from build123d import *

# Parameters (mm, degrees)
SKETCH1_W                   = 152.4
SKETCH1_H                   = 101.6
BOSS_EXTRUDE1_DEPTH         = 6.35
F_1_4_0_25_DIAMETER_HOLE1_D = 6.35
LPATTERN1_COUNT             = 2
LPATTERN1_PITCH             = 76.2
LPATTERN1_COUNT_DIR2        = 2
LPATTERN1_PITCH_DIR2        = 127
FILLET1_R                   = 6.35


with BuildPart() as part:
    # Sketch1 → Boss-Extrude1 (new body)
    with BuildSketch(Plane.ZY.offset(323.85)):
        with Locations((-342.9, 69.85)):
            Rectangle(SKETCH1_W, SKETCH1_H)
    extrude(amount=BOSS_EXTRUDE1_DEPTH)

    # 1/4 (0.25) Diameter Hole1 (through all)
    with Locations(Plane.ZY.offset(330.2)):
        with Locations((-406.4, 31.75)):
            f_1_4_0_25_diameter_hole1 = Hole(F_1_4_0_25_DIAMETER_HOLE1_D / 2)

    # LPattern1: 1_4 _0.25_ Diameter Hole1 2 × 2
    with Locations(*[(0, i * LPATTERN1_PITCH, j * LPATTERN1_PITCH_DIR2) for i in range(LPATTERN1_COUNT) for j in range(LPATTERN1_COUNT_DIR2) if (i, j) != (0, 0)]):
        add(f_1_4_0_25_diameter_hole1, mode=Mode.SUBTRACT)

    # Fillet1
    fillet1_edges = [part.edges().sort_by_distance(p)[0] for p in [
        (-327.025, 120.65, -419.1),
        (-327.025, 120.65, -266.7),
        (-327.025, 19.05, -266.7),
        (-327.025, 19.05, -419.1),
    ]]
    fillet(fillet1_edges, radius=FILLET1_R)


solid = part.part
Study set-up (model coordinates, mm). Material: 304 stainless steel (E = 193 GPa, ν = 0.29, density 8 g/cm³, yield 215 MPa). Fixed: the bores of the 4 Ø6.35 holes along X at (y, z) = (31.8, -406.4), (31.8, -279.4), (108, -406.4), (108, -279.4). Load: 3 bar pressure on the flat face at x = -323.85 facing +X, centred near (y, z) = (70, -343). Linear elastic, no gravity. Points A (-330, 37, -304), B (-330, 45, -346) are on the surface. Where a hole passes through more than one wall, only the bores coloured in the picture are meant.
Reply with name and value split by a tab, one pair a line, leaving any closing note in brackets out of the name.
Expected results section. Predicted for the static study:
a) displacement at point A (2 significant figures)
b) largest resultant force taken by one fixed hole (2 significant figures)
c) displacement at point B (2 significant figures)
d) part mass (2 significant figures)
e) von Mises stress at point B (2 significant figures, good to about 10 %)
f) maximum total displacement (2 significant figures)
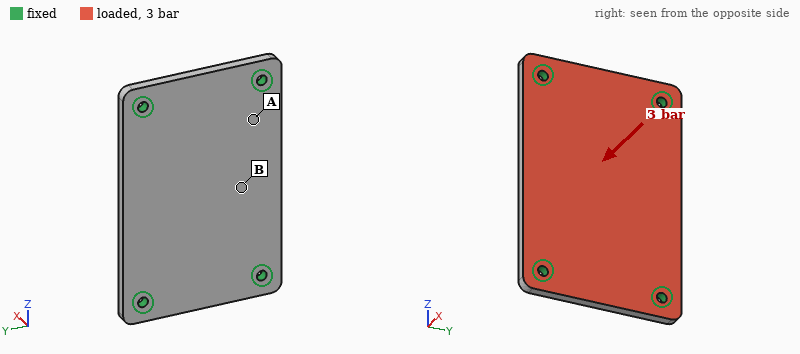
displacement at point A	29 µm
largest resultant force taken by one fixed hole	1.1 kN
displacement at point B	64 µm
part mass	780 g
von Mises stress at point B	31 MPa
maximum total displacement	67 µm
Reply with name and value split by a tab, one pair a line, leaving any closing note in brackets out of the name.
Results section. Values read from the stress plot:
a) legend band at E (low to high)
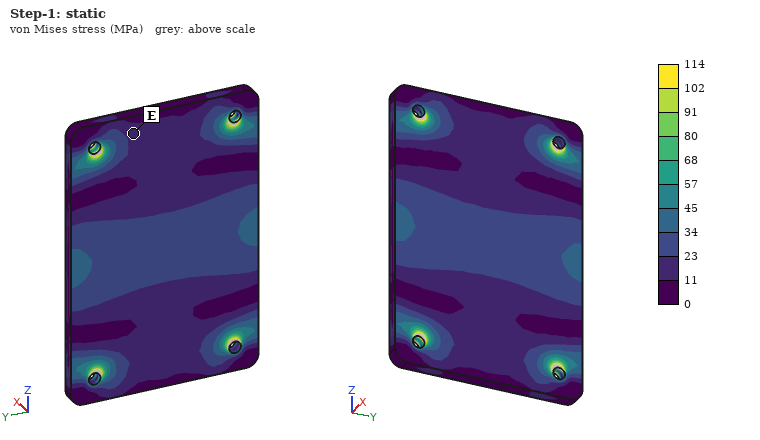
legend band at E	11 to 23 MPa
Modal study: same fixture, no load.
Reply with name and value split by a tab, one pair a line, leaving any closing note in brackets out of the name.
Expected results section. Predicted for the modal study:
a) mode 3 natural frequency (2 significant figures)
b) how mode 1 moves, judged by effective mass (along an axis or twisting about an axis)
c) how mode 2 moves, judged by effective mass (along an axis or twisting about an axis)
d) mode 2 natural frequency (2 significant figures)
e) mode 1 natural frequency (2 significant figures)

mode 3 natural frequency	4300 Hz
how mode 1 moves, judged by effective mass	along X
how mode 2 moves, judged by effective mass	twisting about Z
mode 2 natural frequency	2500 Hz
mode 1 natural frequency	1700 Hz
